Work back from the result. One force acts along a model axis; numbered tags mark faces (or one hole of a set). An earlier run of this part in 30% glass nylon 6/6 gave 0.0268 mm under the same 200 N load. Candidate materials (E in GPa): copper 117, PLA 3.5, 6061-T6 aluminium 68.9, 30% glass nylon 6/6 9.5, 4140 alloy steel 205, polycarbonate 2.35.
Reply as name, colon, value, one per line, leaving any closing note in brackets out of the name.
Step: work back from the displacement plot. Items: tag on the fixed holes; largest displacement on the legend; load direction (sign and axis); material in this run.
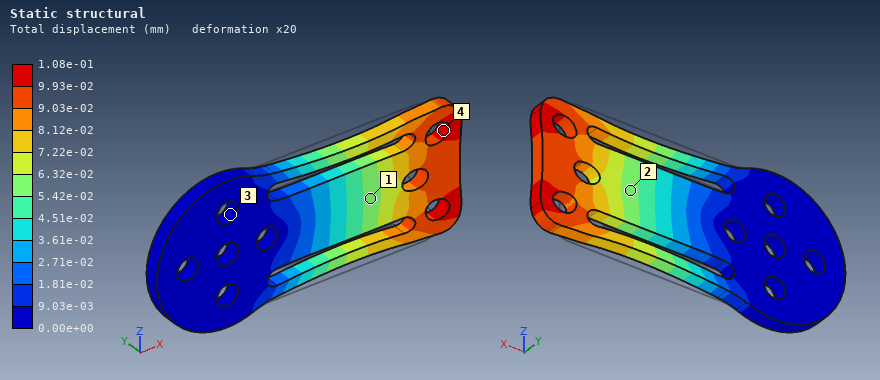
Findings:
tag on the fixed holes: 3
largest displacement on the legend: 1.08e-01 mm
load direction: +X
material in this run: polycarbonate
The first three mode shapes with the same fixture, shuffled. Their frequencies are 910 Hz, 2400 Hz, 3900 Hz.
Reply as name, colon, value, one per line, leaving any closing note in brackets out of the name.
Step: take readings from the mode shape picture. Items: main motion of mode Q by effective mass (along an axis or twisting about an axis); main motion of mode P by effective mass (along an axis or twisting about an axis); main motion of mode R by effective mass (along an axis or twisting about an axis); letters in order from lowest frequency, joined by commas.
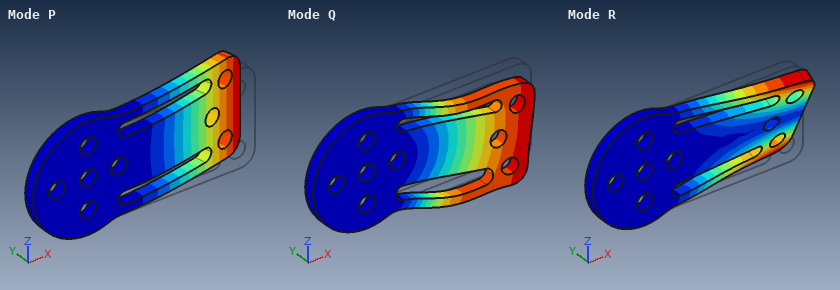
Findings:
main motion of mode Q by effective mass: along Z
main motion of mode P by effective mass: along Y
main motion of mode R by effective mass: twisting about X
letters in order from lowest frequency, joined by commas: P, R, Q
